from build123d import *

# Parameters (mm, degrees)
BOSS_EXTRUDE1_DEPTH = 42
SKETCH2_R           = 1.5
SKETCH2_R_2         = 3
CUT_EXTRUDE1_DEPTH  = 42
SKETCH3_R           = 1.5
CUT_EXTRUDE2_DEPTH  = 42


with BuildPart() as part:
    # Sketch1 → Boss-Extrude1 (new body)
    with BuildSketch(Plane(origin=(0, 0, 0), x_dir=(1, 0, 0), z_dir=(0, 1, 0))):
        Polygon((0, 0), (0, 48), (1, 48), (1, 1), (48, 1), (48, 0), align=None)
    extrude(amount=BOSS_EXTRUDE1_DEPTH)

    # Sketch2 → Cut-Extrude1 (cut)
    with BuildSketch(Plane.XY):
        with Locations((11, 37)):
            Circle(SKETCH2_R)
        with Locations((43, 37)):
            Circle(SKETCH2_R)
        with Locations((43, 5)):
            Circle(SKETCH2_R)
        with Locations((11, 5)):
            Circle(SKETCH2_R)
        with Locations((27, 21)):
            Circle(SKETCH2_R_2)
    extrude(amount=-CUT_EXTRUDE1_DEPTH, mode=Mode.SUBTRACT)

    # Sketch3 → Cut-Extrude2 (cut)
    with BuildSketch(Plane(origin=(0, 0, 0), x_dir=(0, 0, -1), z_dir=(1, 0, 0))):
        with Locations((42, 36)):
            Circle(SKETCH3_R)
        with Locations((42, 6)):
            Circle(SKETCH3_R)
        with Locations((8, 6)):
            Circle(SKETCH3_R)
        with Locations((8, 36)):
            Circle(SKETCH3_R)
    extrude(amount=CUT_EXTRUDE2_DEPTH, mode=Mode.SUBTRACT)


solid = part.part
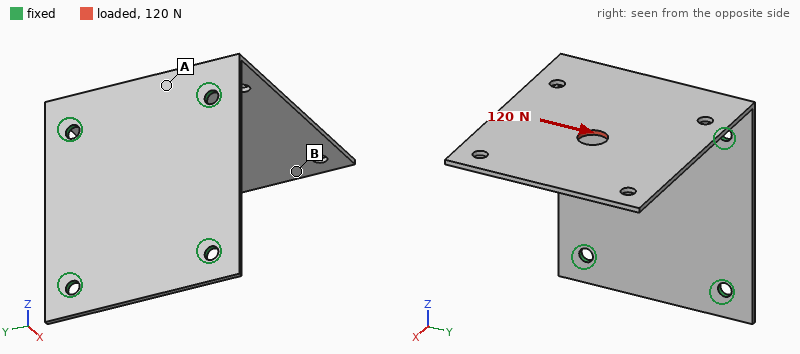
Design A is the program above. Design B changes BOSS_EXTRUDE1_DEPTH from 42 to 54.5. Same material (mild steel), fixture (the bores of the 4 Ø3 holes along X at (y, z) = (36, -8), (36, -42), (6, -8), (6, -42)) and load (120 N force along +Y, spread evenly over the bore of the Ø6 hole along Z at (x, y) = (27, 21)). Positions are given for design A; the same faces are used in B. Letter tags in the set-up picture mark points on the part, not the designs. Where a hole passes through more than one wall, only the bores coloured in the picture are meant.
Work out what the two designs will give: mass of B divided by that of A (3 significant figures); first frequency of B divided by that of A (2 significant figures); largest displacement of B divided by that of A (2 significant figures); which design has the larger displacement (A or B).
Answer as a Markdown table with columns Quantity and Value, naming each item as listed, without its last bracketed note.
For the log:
| Quantity | Value |
|---|---|
| mass of B divided by that of A | 1.30 |
| first frequency of B divided by that of A | 0.98 |
| largest displacement of B divided by that of A | 1.2 |
| which design has the larger displacement | B |
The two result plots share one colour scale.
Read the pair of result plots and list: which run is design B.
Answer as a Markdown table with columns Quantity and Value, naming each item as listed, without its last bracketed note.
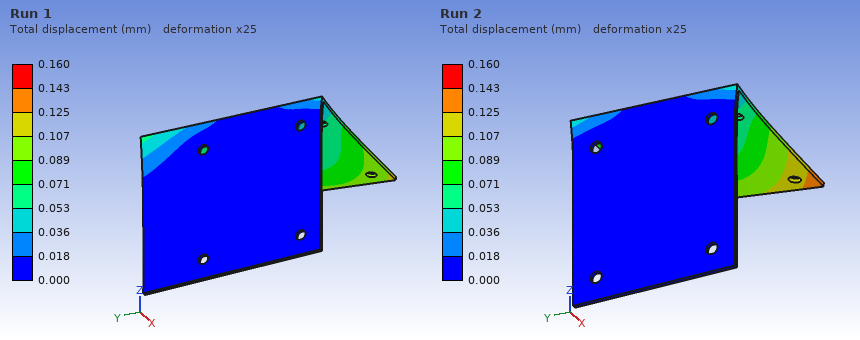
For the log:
| Quantity | Value |
|---|---|
| which run is design B | Run 1 |
